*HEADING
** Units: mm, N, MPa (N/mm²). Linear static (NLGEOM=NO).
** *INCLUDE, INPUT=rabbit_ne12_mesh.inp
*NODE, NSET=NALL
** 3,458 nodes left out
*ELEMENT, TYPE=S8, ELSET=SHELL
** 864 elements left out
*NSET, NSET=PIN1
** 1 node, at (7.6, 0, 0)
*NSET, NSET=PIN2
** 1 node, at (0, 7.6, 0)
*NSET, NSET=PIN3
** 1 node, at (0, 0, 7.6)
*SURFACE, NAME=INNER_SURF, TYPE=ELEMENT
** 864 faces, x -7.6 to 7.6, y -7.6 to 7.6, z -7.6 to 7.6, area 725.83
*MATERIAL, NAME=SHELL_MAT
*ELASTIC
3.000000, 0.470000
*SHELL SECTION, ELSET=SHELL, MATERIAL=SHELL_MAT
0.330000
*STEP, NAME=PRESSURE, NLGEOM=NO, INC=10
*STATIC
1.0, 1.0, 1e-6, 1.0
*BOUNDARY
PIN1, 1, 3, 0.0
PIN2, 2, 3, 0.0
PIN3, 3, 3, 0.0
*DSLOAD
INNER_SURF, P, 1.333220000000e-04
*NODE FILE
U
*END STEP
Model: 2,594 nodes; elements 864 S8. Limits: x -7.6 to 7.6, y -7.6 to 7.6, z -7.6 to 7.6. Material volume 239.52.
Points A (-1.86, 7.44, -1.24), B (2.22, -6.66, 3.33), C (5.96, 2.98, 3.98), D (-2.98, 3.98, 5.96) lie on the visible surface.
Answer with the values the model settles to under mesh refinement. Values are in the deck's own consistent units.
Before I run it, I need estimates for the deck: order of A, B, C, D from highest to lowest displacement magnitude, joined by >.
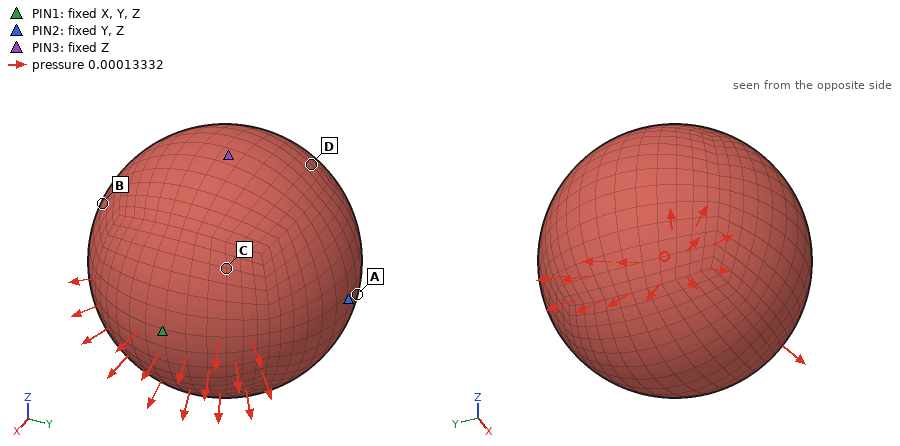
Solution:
D > B > A > C
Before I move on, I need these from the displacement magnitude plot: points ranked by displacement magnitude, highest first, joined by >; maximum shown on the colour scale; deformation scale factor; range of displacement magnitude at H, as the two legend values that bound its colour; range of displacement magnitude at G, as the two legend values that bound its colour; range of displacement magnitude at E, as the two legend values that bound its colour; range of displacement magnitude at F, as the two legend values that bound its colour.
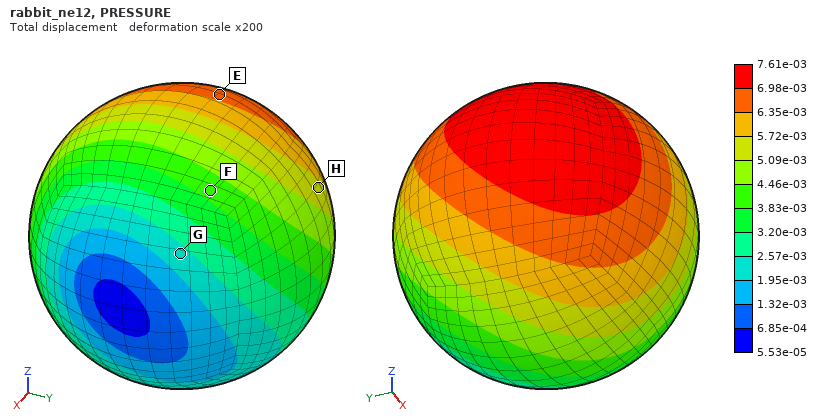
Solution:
E > H > F > G
7.61e-03
200
5.09e-03 to 5.72e-03
1.95e-03 to 2.57e-03
6.35e-03 to 6.98e-03
3.83e-03 to 4.46e-03
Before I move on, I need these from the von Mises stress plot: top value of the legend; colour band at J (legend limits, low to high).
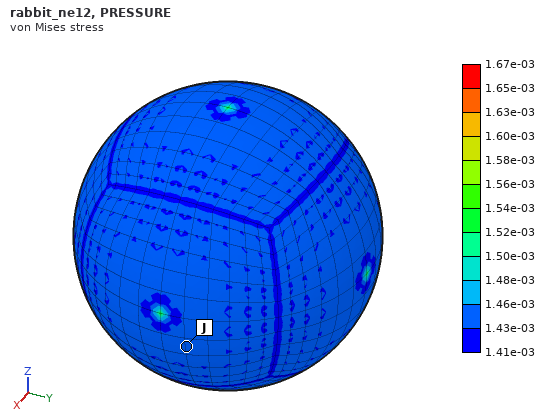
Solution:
1.67e-03
1.43e-03 to 1.46e-03
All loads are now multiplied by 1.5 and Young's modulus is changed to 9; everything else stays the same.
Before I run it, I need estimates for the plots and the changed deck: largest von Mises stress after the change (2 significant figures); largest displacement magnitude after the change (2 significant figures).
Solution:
0.0025
0.0038
